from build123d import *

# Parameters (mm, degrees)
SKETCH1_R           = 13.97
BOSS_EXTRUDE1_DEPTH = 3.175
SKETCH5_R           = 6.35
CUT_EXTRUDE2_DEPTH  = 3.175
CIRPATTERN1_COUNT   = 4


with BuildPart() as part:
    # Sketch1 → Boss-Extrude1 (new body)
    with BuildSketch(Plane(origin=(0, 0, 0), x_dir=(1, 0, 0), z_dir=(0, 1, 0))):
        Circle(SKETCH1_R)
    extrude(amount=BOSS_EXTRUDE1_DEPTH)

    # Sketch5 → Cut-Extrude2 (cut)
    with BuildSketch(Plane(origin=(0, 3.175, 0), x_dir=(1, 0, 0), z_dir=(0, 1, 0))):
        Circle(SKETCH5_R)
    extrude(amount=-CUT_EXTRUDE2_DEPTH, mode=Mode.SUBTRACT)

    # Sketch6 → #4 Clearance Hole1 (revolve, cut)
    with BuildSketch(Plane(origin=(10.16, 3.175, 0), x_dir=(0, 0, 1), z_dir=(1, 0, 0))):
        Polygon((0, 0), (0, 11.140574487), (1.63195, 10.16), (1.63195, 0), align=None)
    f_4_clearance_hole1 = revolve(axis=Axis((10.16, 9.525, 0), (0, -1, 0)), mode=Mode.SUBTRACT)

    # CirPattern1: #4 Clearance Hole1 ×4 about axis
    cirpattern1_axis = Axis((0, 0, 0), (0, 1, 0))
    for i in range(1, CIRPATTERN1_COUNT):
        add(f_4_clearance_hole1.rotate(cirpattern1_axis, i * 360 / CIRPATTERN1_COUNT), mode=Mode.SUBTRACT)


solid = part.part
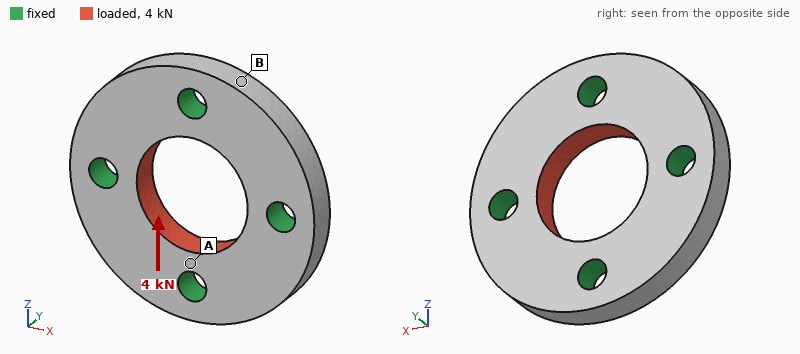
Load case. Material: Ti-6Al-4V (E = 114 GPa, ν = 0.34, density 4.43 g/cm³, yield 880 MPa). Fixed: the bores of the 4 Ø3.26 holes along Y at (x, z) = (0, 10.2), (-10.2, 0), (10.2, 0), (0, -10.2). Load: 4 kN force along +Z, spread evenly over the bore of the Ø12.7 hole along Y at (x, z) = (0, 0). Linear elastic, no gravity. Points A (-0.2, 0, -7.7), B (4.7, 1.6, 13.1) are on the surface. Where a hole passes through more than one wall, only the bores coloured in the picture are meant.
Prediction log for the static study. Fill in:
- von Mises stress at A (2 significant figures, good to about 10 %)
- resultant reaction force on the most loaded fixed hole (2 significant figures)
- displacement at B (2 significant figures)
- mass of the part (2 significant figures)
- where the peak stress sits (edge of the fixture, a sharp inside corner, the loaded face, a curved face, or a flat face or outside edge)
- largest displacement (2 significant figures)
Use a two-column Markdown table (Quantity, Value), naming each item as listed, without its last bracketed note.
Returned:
| Quantity | Value |
|---|---|
| von Mises stress at A | 44 MPa |
| resultant reaction force on the most loaded fixed hole | 1.0 kN |
| displacement at B | 0.99 µm |
| mass of the part | 6.4 g |
| where the peak stress sits | edge of the fixture |
| largest displacement | 2.7 µm |
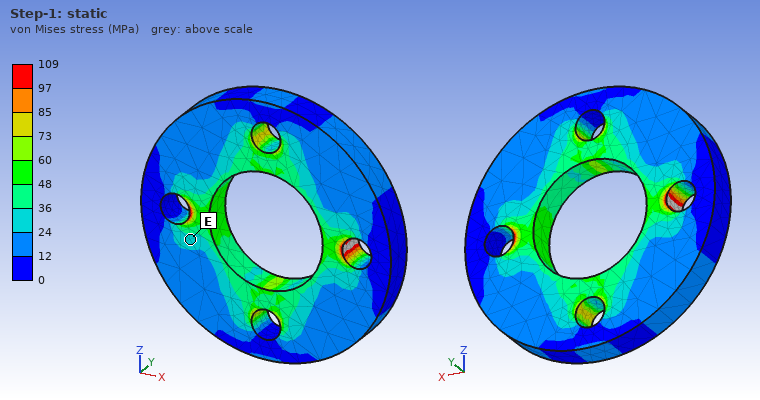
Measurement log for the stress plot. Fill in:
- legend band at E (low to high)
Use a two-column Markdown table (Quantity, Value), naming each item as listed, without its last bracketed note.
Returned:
| Quantity | Value |
|---|---|
| legend band at E | 24 to 36 MPa |
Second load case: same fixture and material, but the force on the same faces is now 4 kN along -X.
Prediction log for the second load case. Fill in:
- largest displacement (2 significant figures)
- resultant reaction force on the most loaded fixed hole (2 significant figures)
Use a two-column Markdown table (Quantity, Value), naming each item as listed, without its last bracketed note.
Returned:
| Quantity | Value |
|---|---|
| largest displacement | 2.7 µm |
| resultant reaction force on the most loaded fixed hole | 1.0 kN |
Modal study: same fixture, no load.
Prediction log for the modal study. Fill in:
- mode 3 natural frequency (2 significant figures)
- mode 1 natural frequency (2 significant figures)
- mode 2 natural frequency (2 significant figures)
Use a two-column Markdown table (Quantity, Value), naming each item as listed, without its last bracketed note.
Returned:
| Quantity | Value |
|---|---|
| mode 3 natural frequency | 52 kHz |
| mode 1 natural frequency | 51 kHz |
| mode 2 natural frequency | 52 kHz |
